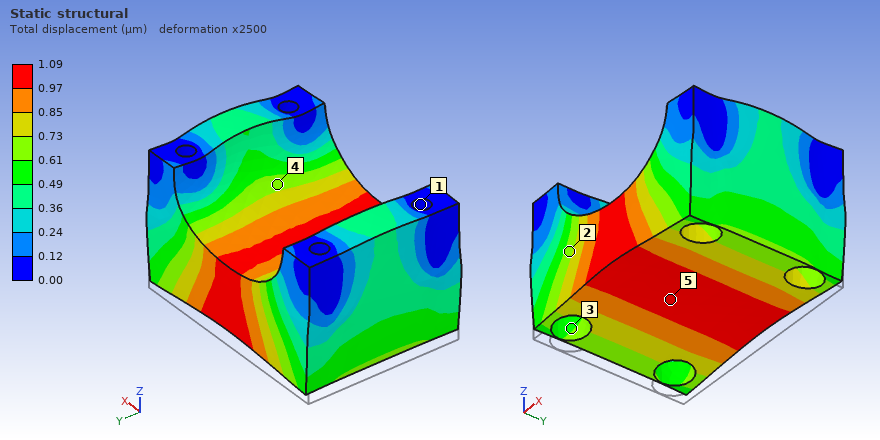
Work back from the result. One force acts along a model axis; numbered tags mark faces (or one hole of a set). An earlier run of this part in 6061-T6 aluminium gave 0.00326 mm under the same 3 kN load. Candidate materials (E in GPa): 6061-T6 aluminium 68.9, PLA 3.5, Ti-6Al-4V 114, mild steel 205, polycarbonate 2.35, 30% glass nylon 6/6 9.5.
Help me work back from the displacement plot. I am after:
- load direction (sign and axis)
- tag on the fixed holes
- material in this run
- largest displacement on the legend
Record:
+Z
1
mild steel
1.09 µm
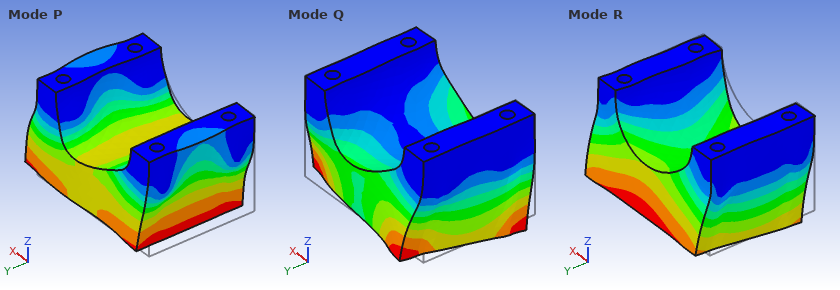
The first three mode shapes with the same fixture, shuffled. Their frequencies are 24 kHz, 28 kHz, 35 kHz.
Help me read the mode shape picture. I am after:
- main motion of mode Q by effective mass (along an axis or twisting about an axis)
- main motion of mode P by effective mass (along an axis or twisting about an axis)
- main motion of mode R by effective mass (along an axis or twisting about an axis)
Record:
twisting about Z
along X
along Y
